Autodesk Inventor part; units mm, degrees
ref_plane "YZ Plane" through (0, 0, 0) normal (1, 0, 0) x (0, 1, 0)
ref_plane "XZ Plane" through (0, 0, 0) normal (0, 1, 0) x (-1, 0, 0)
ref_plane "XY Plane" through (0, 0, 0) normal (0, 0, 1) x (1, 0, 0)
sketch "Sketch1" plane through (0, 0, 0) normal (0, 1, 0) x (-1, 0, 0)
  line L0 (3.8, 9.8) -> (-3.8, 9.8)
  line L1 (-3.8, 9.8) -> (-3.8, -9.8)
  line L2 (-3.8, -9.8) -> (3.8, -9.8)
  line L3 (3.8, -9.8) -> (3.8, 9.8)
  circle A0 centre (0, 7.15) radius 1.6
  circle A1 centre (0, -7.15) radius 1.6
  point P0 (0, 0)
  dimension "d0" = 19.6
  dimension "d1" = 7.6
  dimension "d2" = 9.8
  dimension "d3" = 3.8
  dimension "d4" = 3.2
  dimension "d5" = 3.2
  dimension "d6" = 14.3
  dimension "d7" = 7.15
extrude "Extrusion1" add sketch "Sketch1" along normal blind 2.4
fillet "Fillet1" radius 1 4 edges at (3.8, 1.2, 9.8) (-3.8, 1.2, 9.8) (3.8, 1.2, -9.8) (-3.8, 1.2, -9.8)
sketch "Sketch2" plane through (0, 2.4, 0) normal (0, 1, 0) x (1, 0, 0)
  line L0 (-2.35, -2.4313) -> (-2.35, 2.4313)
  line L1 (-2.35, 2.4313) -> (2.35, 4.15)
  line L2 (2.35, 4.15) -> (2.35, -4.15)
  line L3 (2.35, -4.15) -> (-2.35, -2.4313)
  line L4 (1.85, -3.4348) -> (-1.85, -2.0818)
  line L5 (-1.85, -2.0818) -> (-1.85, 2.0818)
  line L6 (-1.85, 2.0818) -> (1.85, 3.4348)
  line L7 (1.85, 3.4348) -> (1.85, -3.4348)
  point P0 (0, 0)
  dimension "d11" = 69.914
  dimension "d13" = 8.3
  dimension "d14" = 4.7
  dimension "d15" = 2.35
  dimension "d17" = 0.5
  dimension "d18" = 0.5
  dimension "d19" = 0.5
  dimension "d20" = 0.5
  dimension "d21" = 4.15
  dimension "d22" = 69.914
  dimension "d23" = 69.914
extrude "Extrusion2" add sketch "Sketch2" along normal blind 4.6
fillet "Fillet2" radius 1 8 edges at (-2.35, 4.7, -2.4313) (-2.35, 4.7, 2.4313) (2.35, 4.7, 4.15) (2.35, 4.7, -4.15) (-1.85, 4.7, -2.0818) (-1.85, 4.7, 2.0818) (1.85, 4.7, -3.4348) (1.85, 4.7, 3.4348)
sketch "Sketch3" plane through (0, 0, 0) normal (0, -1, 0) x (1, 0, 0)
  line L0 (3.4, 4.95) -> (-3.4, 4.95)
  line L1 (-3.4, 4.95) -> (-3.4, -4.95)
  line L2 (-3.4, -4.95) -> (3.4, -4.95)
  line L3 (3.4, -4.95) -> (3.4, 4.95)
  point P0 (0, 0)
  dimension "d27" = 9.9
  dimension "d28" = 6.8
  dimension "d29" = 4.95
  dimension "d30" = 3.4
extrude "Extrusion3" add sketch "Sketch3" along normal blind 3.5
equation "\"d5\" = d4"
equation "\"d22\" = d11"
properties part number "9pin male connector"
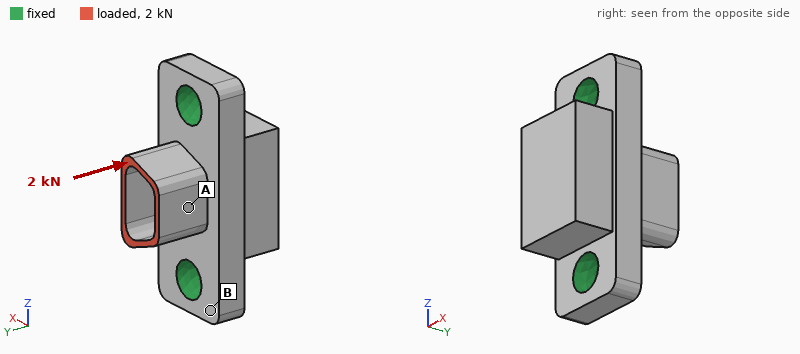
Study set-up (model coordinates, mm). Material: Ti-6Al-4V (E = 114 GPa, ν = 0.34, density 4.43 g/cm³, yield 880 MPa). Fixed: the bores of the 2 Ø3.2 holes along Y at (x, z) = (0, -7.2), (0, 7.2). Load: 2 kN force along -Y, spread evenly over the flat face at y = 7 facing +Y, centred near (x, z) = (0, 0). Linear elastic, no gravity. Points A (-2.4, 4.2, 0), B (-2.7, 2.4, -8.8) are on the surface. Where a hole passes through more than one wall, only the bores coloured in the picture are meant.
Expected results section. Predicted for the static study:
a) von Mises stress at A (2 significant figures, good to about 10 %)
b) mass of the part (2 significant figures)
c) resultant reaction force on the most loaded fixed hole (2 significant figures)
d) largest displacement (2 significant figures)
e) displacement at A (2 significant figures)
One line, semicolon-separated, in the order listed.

160 MPa; 2.7 g; 1.0 kN; 16 µm; 9.7 µm
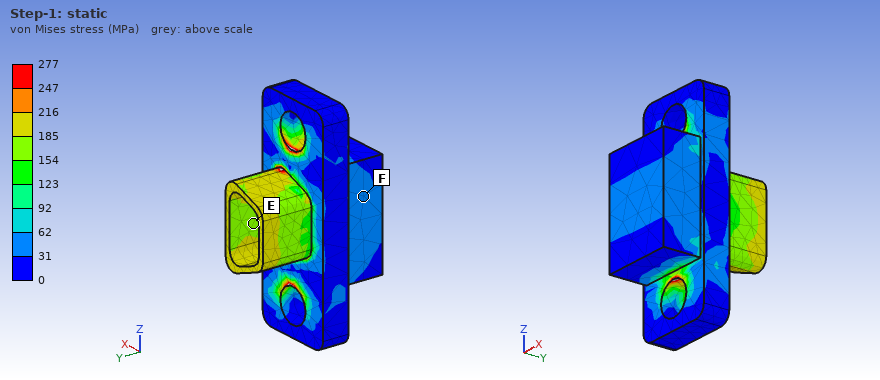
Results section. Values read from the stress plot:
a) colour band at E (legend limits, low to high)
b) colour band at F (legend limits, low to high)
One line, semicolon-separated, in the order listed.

154 to 185 MPa; 31 to 62 MPa
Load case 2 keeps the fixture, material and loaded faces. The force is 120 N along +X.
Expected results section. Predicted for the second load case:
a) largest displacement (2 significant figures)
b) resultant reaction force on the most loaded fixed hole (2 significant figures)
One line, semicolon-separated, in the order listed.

24 µm; 60 N
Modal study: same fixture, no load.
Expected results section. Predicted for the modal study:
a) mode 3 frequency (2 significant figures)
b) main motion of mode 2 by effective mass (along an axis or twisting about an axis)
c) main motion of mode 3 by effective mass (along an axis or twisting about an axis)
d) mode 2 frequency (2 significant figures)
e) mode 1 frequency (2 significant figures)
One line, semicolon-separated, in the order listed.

65 kHz; along X; along Y; 57 kHz; 41 kHz
